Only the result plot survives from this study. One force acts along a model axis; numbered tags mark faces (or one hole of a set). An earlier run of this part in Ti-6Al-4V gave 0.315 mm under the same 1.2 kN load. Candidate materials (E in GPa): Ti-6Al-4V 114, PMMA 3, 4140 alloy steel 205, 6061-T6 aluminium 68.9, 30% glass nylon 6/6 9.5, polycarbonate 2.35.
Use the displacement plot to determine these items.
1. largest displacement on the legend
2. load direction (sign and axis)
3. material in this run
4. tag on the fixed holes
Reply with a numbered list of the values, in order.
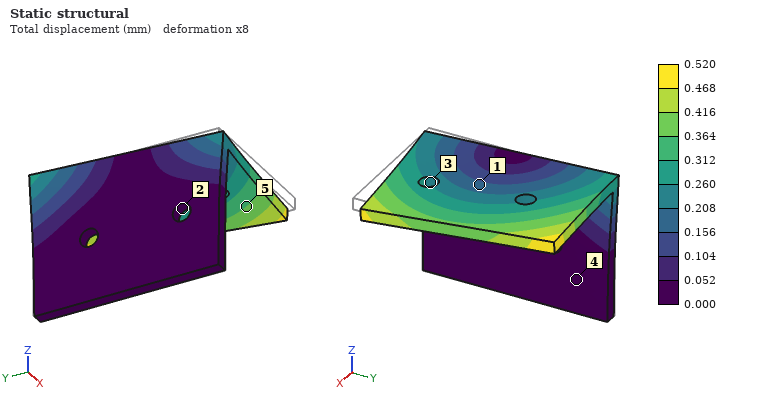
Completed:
1. 0.520 mm
2. +Y
3. 6061-T6 aluminium
4. 2
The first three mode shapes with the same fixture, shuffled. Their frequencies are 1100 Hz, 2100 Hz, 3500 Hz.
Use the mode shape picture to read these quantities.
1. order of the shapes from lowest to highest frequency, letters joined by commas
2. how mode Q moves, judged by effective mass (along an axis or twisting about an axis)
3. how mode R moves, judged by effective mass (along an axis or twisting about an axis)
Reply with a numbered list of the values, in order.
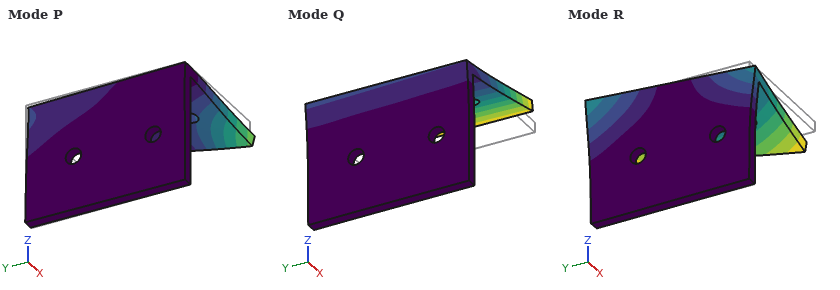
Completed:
1. Q, R, P
2. along Z
3. along Y
